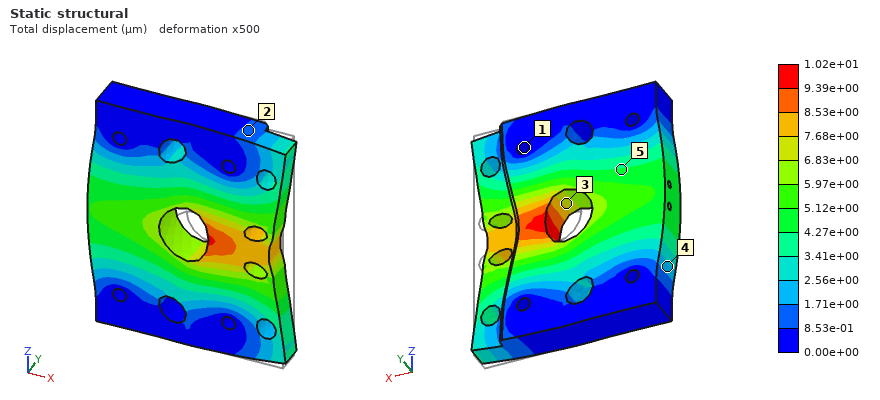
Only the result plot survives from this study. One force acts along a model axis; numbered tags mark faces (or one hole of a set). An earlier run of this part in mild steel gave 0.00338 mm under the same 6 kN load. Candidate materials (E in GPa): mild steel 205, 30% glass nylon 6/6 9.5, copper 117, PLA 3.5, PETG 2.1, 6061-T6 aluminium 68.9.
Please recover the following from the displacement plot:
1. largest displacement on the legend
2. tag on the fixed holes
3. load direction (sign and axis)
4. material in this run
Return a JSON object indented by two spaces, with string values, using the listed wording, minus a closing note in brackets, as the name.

{
  "largest displacement on the legend": "1.02e+01 µm",
  "tag on the fixed holes": "1",
  "load direction": "-X",
  "material in this run": "6061-T6 aluminium"
}
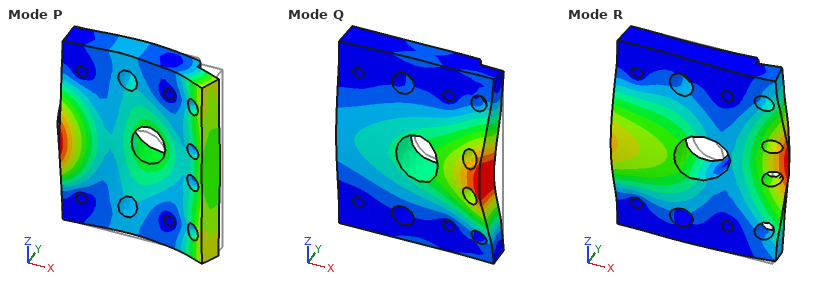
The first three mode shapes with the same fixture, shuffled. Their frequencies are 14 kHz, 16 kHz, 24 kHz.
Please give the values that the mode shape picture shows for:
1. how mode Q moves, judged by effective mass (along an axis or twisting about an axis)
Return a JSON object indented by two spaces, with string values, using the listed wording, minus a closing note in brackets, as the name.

{
  "how mode Q moves, judged by effective mass": "along Y"
}
